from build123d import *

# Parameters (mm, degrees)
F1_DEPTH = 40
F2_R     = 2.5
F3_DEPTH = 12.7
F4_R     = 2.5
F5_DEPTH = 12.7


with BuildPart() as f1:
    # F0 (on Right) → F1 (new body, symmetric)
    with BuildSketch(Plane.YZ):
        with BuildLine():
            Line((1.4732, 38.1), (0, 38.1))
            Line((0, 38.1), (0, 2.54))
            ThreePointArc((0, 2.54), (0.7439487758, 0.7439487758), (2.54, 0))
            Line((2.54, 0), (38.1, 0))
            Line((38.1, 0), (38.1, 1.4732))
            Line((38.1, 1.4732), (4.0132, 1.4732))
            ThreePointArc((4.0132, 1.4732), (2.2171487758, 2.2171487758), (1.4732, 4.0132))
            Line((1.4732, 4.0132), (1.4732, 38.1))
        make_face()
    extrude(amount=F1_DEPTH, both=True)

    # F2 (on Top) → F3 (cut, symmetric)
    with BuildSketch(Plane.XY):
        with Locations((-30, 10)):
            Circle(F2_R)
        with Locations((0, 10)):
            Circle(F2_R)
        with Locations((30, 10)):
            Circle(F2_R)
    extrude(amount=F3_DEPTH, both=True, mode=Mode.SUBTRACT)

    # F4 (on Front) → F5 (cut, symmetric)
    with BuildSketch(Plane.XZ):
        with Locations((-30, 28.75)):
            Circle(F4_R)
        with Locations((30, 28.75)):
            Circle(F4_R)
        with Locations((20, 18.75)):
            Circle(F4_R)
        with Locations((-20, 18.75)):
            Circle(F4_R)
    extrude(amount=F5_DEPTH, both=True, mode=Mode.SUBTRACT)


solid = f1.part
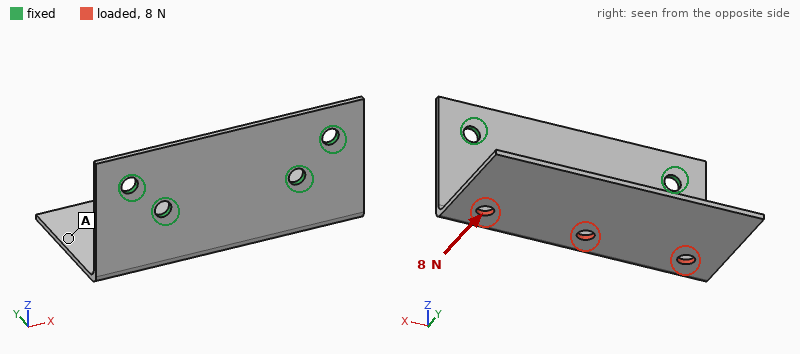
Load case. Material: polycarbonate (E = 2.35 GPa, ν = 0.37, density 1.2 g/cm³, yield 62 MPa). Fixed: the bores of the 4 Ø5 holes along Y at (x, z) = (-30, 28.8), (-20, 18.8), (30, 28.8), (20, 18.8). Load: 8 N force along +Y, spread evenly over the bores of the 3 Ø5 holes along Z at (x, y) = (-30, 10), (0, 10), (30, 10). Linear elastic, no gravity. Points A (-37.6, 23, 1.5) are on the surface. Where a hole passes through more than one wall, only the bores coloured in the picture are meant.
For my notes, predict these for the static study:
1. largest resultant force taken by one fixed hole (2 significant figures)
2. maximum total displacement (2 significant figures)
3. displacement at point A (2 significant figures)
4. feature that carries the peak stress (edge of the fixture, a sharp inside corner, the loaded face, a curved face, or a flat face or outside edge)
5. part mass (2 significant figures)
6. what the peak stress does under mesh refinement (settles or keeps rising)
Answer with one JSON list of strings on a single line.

["5.2 N", "0.96 mm", "0.61 mm", "edge of the fixture", "10 g", "keeps rising"]
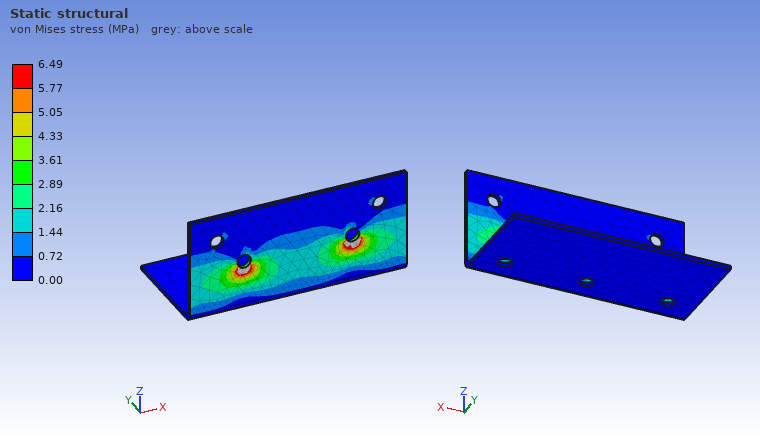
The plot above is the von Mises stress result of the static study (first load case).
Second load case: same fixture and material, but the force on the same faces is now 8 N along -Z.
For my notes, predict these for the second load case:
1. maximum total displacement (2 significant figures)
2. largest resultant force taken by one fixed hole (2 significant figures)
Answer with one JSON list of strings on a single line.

["1.0 mm", "2.9 N"]
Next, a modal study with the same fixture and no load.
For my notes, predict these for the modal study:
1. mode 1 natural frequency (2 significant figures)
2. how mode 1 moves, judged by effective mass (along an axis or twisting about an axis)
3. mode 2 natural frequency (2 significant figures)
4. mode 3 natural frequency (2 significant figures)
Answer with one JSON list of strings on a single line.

["140 Hz", "along Z", "240 Hz", "420 Hz"]
